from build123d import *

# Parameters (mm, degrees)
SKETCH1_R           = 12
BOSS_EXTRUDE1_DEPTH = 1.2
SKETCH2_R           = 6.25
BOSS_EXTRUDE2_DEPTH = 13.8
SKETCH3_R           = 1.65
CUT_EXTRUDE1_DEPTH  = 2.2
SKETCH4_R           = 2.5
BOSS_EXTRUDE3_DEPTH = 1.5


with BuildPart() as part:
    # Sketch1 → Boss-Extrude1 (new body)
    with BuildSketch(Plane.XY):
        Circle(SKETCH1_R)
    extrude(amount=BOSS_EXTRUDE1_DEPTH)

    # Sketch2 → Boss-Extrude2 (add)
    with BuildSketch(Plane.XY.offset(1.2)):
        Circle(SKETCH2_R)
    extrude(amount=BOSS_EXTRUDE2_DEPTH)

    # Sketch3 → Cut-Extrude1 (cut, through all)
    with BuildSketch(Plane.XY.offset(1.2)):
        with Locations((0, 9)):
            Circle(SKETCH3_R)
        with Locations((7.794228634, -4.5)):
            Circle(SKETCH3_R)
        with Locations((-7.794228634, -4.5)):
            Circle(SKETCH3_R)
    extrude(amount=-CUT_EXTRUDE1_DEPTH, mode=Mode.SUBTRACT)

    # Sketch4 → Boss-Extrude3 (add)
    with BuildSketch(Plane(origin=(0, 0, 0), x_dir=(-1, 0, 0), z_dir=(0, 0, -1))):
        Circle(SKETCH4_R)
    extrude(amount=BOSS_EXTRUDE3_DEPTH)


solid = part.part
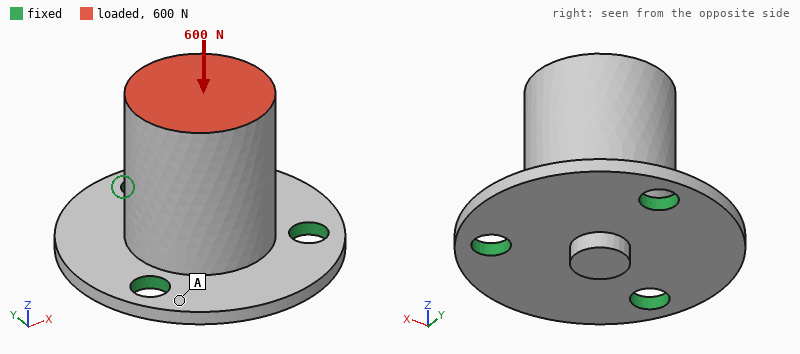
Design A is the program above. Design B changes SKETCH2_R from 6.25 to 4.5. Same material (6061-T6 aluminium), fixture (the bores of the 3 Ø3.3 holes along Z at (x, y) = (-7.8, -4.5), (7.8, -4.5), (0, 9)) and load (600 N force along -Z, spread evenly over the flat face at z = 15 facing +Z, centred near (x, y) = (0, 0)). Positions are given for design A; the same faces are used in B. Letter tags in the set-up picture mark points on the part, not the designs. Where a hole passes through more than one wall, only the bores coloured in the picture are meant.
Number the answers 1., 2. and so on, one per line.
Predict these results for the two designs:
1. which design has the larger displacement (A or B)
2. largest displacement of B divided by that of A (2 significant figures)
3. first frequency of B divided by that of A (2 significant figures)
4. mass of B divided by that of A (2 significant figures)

1. B
2. 3.0
3. 0.74
4. 0.64
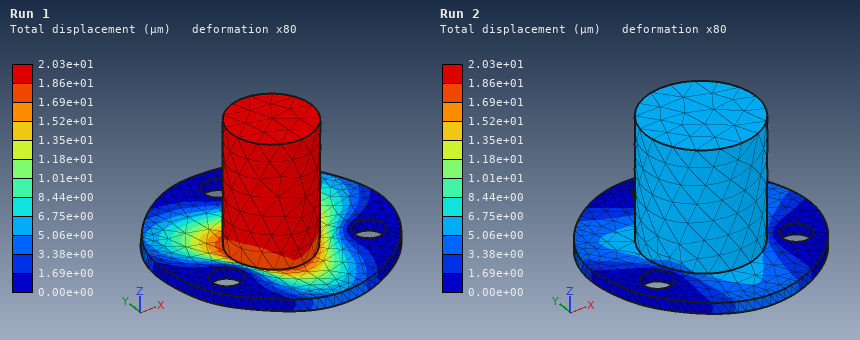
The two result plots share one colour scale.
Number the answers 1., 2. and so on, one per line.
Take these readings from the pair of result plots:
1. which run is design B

1. Run 1
